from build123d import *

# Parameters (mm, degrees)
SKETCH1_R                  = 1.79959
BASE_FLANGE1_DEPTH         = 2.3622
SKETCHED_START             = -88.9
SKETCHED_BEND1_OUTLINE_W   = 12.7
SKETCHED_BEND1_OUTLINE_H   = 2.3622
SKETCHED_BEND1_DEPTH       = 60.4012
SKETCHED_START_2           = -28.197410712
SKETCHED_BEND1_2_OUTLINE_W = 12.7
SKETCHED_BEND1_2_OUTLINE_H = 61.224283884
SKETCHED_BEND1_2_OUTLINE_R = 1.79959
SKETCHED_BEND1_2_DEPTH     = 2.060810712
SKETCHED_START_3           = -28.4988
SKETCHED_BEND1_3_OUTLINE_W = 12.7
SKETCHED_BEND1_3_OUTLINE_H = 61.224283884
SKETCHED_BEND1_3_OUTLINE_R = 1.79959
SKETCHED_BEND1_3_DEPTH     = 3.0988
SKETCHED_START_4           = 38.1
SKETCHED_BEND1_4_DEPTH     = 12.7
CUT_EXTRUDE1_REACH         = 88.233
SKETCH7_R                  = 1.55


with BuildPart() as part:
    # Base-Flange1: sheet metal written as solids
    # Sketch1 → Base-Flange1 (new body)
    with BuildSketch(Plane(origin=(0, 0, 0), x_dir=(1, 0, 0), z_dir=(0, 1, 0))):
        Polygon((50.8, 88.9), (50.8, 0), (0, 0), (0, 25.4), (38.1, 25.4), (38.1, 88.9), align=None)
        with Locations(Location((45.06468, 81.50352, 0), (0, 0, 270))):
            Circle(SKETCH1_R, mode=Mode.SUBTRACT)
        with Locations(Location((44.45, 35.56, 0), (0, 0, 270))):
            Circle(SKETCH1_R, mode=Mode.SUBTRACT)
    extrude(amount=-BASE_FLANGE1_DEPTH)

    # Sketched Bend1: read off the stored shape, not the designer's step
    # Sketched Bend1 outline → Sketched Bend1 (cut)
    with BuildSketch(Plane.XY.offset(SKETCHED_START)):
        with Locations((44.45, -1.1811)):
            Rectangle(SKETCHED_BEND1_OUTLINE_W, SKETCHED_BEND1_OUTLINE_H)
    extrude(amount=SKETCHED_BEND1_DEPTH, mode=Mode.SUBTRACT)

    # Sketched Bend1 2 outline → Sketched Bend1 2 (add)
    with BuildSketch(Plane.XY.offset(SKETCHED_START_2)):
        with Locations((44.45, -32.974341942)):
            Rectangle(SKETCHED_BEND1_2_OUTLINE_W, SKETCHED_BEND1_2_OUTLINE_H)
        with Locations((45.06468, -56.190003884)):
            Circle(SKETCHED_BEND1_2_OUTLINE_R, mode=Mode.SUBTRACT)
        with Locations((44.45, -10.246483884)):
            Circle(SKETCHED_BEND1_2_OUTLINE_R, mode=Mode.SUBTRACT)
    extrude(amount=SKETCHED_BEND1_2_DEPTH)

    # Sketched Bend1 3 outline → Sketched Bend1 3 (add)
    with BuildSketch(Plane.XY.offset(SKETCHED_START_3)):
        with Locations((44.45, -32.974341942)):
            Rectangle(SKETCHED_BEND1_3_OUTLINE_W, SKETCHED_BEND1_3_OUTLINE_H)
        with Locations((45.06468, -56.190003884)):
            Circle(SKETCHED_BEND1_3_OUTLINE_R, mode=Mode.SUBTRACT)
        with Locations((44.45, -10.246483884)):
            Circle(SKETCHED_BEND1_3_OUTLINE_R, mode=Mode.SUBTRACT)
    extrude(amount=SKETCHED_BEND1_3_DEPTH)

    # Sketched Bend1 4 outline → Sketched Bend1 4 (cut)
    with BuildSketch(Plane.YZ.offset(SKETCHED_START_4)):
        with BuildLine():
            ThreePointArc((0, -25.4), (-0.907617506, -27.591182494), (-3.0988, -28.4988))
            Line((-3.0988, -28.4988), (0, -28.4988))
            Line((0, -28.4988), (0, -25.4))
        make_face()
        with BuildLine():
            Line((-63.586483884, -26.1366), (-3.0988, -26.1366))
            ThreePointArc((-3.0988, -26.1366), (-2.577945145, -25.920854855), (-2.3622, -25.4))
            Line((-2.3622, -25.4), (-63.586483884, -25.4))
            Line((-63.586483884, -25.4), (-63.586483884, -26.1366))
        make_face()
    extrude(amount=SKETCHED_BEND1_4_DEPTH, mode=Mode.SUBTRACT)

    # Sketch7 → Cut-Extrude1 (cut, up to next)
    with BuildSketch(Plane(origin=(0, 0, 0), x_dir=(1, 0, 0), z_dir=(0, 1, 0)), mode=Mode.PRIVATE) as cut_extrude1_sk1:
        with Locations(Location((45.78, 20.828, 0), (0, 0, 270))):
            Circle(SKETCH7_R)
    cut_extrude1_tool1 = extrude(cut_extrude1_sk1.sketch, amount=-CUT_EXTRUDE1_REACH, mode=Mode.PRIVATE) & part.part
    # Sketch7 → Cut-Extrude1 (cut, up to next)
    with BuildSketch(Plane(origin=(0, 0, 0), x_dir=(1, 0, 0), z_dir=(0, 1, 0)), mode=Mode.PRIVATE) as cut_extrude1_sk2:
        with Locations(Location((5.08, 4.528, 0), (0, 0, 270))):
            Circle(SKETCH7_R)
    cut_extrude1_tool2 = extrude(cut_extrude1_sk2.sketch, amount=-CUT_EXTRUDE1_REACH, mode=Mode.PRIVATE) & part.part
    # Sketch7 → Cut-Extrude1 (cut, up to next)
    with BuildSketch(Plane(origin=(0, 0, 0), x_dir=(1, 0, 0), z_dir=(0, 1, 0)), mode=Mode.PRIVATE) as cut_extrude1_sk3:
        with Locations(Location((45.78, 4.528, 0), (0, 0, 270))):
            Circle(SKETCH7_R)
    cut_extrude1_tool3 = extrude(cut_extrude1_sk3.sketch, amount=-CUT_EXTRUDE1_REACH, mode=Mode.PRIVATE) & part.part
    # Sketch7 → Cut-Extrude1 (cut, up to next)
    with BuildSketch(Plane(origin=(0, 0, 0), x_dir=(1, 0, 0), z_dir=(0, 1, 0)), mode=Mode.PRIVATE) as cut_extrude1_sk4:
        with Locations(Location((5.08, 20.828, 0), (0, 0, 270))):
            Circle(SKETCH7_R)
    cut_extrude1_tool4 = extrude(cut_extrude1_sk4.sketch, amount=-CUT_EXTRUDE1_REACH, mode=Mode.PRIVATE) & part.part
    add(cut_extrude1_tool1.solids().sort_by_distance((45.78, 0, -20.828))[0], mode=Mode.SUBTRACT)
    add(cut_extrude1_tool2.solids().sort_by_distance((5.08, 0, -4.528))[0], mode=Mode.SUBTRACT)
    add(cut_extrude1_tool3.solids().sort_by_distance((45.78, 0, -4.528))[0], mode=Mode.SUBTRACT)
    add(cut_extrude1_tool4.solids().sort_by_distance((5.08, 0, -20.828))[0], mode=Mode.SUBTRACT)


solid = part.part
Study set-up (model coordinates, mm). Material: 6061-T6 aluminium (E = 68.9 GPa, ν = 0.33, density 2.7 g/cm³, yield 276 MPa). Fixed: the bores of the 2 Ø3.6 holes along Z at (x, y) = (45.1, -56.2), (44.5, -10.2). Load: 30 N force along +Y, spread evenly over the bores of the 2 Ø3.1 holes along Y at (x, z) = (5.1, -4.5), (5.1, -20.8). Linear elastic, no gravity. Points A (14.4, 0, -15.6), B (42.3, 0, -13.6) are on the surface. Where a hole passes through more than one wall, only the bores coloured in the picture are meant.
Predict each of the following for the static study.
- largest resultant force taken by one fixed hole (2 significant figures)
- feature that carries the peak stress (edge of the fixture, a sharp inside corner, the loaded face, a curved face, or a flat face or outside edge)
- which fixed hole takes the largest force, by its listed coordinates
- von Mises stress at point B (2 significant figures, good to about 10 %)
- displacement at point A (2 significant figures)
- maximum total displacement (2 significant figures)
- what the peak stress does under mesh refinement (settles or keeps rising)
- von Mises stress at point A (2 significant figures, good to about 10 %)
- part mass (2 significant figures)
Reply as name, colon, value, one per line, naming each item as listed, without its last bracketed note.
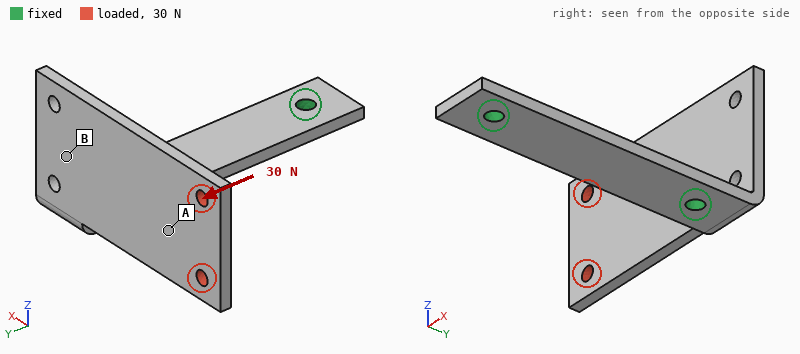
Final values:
largest resultant force taken by one fixed hole: 30 N
feature that carries the peak stress: a sharp inside corner
which fixed hole takes the largest force, by its listed coordinates: (44.5, -10.2)
von Mises stress at point B: 37 MPa
displacement at point A: 0.42 mm
maximum total displacement: 0.81 mm
what the peak stress does under mesh refinement: keeps rising
von Mises stress at point A: 12 MPa
part mass: 13 g
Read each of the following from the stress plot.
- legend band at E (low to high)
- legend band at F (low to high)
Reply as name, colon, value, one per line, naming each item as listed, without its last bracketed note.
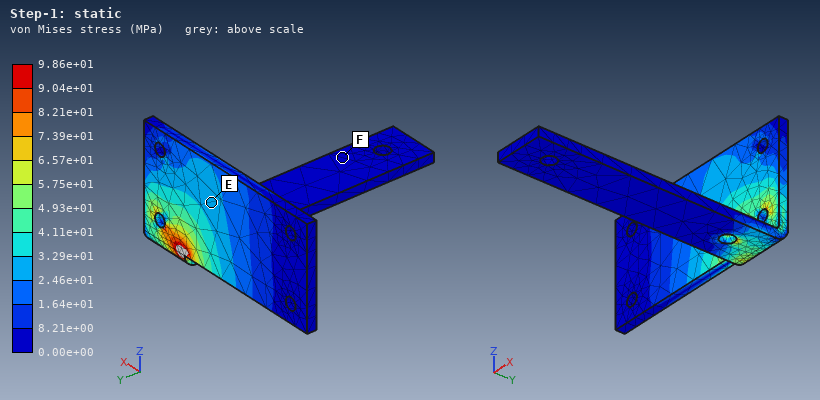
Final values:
legend band at E: 2.46e+01 to 3.29e+01 MPa
legend band at F: 0.00e+00 to 8.21e+00 MPa
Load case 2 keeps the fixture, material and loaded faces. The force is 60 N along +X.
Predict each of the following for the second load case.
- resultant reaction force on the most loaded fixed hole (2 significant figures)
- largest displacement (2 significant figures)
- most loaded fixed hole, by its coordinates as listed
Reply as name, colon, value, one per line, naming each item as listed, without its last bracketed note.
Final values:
resultant reaction force on the most loaded fixed hole: 65 N
largest displacement: 0.23 mm
most loaded fixed hole, by its coordinates as listed: (44.5, -10.2)
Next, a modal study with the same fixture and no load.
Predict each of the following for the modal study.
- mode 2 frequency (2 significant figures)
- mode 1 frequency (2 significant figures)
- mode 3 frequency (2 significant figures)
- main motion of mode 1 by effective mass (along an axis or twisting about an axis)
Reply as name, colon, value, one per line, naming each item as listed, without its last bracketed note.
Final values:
mode 2 frequency: 900 Hz
mode 1 frequency: 620 Hz
mode 3 frequency: 1400 Hz
main motion of mode 1 by effective mass: along Y
